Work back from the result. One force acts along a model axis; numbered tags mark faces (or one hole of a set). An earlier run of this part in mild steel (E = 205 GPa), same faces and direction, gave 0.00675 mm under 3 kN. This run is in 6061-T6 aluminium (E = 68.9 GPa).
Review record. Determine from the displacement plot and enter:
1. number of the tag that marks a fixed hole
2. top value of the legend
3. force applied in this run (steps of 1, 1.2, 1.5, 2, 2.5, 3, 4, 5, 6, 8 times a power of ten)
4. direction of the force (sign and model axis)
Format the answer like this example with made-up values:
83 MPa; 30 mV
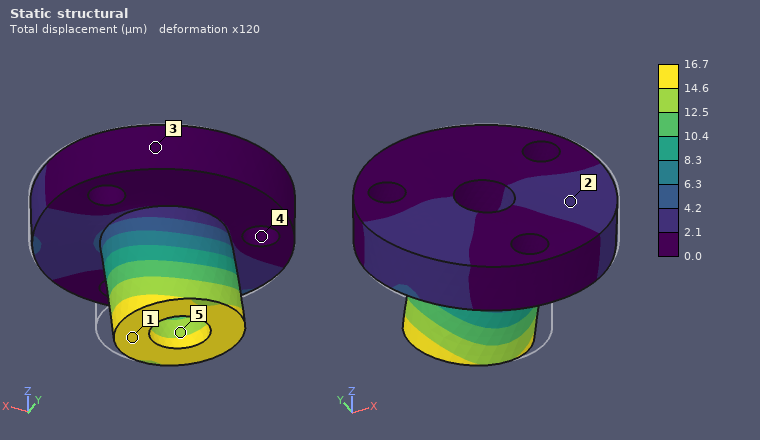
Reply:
4; 16.7 µm; 2.5 kN; -X
